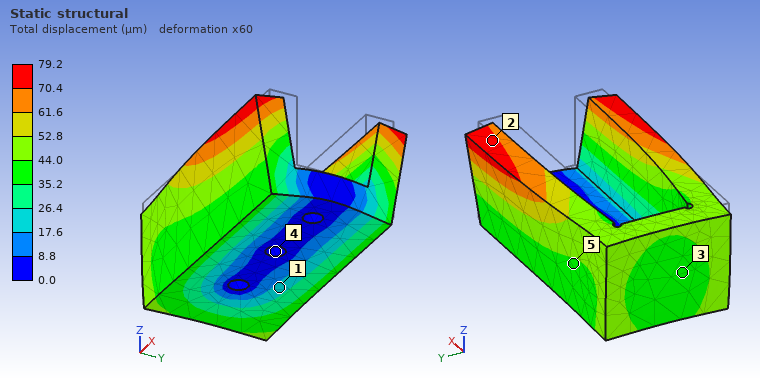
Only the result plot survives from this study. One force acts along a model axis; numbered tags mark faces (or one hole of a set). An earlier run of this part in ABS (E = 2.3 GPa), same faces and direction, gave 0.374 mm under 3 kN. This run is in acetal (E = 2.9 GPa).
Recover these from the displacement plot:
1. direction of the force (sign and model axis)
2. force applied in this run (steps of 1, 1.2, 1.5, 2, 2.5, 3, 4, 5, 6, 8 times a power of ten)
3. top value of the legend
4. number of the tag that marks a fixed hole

-Z
800 N
79.2 µm
4
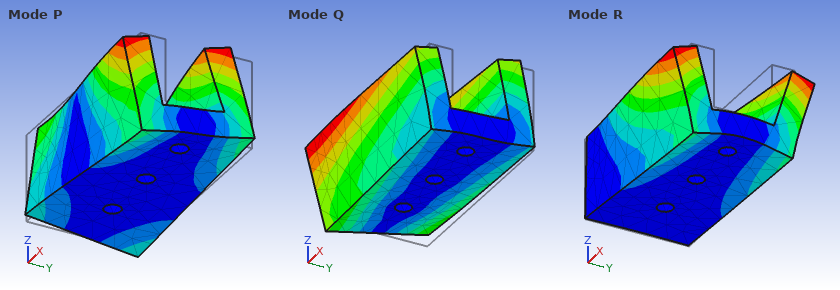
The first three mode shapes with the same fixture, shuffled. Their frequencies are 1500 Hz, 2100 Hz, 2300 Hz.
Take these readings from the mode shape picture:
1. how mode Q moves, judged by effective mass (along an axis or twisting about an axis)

along Y
